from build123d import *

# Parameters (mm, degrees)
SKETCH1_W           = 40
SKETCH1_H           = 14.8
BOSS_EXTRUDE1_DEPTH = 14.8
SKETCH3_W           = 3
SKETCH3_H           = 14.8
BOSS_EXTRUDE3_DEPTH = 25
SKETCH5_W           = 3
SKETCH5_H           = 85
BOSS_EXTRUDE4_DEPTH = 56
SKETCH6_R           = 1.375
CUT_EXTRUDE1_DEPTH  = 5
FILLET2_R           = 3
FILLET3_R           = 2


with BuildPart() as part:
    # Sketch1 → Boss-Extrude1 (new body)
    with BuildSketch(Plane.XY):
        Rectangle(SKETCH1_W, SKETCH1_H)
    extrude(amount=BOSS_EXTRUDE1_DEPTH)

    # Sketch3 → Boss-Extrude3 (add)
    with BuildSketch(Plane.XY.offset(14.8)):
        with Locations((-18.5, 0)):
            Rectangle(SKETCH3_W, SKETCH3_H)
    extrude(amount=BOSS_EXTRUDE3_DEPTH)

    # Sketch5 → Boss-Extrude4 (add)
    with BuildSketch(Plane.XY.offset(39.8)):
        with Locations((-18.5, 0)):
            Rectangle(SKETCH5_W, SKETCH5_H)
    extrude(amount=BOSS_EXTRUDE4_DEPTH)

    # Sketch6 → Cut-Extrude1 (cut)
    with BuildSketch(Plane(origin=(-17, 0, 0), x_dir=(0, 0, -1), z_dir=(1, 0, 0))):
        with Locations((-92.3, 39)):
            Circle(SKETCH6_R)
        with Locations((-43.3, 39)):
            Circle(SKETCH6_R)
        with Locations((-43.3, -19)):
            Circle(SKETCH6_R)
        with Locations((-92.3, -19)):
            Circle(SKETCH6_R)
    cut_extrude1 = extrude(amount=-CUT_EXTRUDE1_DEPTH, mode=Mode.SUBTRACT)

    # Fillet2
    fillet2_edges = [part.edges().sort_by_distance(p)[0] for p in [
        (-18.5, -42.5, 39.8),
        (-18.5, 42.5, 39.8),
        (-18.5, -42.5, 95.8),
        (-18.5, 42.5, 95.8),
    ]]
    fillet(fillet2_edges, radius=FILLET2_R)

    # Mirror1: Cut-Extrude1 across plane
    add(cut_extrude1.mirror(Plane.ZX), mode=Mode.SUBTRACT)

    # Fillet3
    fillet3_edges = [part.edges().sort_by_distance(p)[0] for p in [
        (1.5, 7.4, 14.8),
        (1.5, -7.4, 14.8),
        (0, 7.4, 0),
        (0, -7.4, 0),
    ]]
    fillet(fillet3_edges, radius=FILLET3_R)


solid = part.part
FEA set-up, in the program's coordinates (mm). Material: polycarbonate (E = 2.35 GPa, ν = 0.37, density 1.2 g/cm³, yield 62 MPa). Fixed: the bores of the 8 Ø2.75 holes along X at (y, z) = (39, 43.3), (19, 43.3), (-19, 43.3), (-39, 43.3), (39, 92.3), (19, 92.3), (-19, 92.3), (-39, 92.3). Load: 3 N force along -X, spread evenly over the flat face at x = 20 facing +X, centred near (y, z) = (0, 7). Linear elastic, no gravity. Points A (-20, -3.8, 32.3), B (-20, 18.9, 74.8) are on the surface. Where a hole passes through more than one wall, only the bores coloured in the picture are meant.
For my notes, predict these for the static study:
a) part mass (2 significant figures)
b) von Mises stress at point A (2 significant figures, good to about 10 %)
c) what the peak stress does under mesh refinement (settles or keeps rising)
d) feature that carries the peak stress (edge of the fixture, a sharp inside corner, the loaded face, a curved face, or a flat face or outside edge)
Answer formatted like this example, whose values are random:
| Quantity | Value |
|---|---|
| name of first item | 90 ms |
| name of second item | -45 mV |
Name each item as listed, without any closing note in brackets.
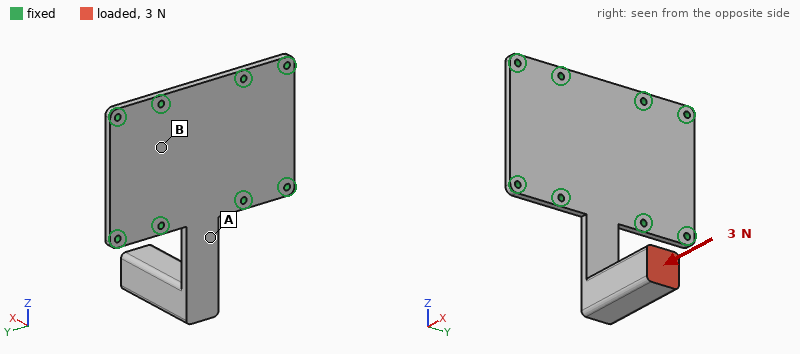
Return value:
| Quantity | Value |
|---|---|
| part mass | 29 g |
| von Mises stress at point A | 3.4 MPa |
| what the peak stress does under mesh refinement | keeps rising |
| feature that carries the peak stress | a sharp inside corner |
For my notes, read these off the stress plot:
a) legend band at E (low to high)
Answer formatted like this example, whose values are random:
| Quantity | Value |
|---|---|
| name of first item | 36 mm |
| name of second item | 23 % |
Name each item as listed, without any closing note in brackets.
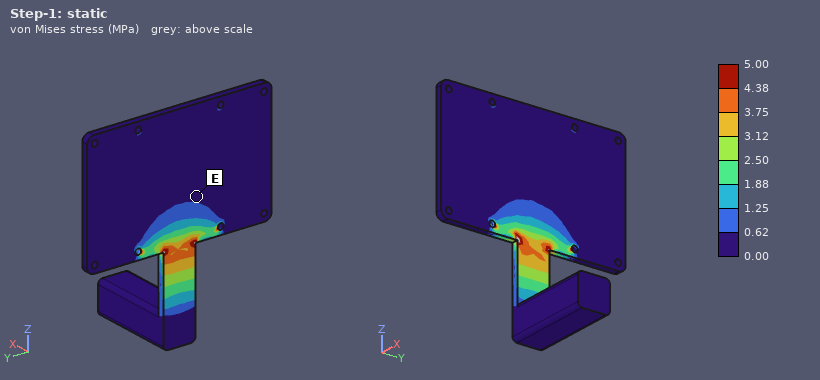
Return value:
| Quantity | Value |
|---|---|
| legend band at E | 0.00 to 0.62 MPa |
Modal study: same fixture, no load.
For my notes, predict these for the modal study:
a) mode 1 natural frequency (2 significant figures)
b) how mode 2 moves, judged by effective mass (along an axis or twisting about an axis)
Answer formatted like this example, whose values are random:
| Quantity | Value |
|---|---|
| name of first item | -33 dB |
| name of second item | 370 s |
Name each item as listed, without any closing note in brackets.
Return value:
| Quantity | Value |
|---|---|
| mode 1 natural frequency | 73 Hz |
| how mode 2 moves, judged by effective mass | along Y |
